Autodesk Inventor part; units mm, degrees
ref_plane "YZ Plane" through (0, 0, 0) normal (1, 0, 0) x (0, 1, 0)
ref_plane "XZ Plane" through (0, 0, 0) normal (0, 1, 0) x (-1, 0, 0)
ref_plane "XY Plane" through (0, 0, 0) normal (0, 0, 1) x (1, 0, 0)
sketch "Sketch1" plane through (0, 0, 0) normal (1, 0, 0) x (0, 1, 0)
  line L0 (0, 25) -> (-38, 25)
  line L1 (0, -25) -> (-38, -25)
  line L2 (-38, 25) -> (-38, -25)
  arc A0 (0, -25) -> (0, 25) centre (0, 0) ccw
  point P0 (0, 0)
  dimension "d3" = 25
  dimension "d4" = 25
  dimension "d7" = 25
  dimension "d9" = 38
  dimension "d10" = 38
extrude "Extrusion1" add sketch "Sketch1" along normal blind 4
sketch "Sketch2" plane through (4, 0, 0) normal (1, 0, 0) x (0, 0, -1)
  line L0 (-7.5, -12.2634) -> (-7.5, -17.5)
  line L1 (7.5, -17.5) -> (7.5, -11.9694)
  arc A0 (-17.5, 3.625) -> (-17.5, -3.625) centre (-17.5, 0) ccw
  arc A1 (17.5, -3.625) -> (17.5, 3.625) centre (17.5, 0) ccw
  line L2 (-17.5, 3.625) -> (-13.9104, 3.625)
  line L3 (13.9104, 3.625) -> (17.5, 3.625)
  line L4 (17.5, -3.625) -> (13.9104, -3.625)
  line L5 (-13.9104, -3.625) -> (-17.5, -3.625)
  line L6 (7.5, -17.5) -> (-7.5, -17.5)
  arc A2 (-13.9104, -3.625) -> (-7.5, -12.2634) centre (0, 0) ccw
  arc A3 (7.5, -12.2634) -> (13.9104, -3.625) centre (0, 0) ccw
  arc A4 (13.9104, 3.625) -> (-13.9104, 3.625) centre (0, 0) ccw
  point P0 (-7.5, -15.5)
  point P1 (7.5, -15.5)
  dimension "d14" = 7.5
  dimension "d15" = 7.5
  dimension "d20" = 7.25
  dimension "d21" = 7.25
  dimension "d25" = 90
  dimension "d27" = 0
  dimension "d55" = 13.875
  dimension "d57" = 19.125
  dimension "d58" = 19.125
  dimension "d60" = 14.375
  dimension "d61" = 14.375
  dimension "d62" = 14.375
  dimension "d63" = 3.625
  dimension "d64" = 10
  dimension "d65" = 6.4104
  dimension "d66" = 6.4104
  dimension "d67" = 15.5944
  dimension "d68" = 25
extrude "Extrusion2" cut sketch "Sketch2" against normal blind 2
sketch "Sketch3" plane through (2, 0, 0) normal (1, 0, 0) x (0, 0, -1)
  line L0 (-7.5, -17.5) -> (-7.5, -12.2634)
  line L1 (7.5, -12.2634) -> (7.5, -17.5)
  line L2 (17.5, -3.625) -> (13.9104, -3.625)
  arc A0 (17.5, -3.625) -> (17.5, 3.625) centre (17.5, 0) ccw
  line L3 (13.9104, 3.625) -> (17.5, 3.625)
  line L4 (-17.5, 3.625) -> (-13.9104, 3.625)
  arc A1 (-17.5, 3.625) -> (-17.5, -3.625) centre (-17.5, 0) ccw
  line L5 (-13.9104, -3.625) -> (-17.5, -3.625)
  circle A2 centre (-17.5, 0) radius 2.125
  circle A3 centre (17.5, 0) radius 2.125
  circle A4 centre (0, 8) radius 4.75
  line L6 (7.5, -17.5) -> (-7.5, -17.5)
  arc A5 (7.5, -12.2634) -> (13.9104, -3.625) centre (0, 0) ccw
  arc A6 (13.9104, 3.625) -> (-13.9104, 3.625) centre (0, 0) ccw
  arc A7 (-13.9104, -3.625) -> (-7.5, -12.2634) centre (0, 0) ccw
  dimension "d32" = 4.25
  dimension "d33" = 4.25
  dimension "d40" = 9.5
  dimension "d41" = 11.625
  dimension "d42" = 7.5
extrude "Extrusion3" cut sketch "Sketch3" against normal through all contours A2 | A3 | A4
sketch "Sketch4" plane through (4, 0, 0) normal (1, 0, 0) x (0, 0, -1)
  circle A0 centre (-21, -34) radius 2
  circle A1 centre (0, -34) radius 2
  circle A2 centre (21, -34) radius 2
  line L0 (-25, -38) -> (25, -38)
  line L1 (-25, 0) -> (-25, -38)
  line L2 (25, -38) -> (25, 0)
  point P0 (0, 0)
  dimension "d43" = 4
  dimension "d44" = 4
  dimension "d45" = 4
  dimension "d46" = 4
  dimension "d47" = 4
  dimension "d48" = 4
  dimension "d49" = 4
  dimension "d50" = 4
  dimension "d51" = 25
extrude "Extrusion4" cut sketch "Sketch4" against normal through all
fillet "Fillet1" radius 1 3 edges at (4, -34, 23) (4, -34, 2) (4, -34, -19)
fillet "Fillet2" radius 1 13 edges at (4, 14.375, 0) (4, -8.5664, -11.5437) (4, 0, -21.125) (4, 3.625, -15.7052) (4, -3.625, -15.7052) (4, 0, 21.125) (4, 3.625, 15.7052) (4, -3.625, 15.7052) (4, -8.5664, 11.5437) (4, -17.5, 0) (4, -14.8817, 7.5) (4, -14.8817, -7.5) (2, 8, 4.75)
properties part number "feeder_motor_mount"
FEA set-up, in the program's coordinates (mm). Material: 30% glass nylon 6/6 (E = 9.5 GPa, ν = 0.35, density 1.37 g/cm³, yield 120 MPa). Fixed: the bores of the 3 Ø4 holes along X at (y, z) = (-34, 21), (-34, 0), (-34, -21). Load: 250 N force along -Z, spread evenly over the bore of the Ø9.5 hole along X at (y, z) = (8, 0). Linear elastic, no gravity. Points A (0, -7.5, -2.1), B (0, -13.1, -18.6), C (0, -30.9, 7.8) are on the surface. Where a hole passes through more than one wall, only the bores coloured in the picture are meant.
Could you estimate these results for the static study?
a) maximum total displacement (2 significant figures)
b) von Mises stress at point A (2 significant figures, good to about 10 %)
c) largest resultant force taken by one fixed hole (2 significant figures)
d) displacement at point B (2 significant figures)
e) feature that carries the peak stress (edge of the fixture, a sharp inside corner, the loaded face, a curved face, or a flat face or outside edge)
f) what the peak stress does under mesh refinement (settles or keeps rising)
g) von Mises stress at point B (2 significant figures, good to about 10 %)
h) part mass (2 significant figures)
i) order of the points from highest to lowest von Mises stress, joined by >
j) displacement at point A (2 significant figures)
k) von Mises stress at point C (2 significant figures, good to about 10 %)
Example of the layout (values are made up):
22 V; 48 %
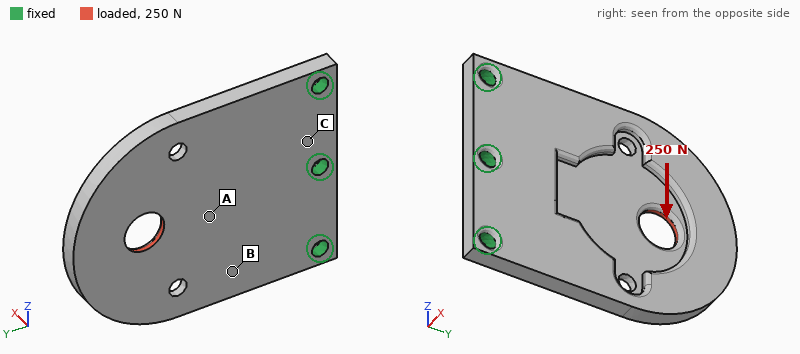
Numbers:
63 µm; 6.5 MPa; 250 N; 23 µm; edge of the fixture; keeps rising; 4.2 MPa; 13 g; A > B > C; 23 µm; 1.9 MPa
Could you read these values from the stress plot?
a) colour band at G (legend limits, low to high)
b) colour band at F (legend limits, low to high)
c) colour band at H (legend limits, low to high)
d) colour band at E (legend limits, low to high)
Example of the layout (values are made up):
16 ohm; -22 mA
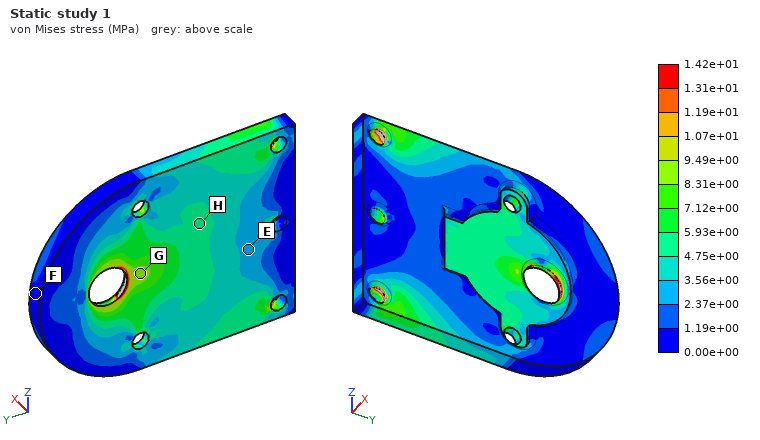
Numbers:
8.31e+00 to 9.49e+00 MPa; 0.00e+00 to 1.19e+00 MPa; 4.75e+00 to 5.93e+00 MPa; 2.37e+00 to 3.56e+00 MPa
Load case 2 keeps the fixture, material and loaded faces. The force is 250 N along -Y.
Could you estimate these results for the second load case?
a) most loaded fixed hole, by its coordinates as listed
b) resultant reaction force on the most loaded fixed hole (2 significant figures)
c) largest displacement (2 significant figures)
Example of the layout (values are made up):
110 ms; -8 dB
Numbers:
(-34, 0); 94 N; 0.26 mm
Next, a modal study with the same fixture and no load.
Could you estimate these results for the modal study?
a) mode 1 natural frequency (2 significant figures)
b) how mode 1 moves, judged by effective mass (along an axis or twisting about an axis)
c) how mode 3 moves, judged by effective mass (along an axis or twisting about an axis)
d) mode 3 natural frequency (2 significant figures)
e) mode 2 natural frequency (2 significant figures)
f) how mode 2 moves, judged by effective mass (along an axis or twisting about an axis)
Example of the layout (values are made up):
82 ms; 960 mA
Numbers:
560 Hz; along X; along X; 2500 Hz; 1500 Hz; twisting about Y
